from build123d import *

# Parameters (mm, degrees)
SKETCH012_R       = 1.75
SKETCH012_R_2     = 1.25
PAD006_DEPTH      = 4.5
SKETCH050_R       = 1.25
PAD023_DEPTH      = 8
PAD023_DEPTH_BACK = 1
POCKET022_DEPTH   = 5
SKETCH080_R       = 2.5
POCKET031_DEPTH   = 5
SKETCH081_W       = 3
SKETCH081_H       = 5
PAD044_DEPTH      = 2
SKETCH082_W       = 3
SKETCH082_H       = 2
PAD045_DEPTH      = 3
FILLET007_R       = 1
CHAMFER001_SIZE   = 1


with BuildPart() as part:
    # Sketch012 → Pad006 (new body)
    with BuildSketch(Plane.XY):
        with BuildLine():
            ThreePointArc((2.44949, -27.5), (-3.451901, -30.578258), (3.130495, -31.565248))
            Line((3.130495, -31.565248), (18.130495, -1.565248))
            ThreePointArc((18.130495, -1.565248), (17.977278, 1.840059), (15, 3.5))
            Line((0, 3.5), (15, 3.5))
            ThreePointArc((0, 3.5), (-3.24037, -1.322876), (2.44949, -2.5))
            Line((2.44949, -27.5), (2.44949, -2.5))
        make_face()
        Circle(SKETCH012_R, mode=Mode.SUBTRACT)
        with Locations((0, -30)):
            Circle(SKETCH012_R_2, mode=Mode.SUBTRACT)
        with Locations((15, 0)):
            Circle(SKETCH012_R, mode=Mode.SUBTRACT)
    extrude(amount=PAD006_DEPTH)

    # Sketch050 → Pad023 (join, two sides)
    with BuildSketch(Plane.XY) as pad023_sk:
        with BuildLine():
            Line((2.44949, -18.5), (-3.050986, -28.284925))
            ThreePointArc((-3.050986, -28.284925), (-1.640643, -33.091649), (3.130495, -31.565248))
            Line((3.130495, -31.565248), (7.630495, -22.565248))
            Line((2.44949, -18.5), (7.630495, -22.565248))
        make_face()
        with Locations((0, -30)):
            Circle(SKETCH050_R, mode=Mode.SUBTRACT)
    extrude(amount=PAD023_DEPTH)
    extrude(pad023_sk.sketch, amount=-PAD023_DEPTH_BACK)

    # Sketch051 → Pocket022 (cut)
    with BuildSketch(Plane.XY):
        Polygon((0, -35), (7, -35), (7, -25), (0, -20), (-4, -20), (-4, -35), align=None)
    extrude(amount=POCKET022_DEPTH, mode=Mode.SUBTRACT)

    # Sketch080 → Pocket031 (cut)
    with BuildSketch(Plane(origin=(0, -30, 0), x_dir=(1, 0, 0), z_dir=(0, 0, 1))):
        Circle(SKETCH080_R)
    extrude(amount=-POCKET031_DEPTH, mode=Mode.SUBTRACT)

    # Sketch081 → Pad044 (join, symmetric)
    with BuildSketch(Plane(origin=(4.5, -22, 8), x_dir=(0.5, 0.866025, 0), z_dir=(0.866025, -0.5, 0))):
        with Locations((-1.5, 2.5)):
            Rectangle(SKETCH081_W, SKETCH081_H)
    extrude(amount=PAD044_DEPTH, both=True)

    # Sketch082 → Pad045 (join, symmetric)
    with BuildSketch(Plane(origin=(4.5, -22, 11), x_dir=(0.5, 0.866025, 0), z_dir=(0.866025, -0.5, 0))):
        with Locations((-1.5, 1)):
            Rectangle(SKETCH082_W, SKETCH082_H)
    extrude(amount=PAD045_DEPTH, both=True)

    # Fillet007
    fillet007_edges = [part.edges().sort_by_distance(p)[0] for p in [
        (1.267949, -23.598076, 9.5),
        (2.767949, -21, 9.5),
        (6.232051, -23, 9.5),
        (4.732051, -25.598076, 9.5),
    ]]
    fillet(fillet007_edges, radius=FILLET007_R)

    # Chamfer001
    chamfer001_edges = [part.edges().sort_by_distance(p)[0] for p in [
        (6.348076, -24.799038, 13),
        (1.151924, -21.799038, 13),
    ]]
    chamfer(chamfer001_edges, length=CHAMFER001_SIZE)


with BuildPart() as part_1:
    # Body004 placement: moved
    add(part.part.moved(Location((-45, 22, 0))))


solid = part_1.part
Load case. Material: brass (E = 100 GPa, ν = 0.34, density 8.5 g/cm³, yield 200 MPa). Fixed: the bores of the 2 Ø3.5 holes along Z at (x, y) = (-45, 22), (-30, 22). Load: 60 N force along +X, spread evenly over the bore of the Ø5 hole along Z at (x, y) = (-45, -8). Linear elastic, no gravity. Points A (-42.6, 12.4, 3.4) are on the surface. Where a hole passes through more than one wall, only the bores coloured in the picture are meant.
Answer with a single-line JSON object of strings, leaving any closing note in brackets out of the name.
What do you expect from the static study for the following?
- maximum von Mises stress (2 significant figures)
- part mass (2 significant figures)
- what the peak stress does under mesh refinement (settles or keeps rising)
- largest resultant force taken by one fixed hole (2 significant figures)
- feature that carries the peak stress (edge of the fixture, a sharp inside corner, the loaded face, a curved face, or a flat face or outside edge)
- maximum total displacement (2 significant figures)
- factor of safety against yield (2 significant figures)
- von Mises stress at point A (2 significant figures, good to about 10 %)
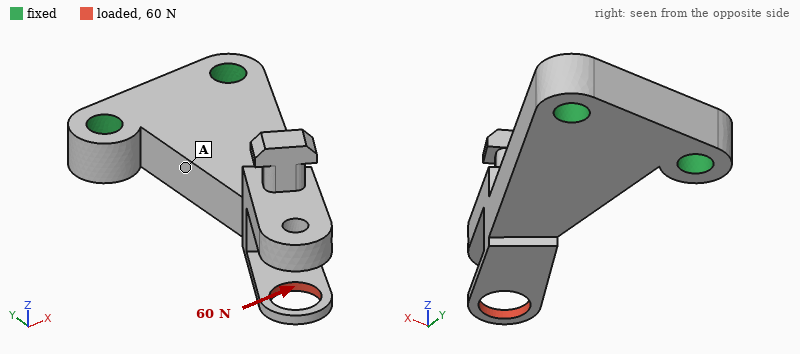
{"maximum von Mises stress": "100 MPa", "part mass": "16 g", "what the peak stress does under mesh refinement": "settles", "largest resultant force taken by one fixed hole": "130 N", "feature that carries the peak stress": "the loaded face", "maximum total displacement": "43 µm", "factor of safety against yield": "1.9", "von Mises stress at point A": "14 MPa"}
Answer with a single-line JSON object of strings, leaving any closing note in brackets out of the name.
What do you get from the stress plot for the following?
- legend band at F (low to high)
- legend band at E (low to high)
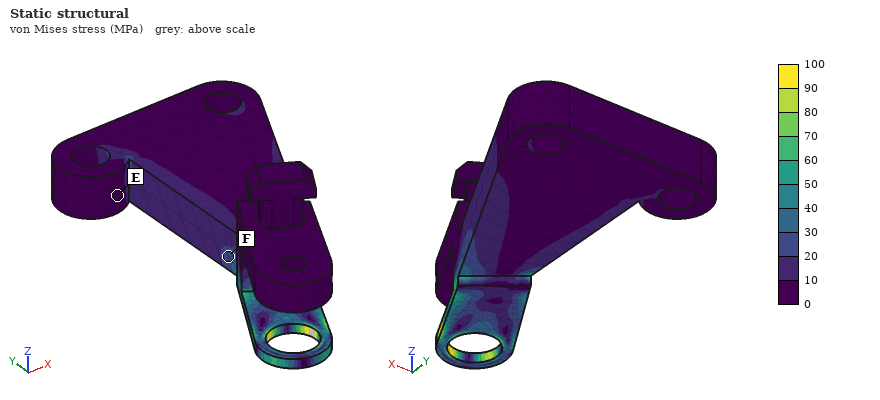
{"legend band at F": "20 to 30 MPa", "legend band at E": "0 to 10 MPa"}
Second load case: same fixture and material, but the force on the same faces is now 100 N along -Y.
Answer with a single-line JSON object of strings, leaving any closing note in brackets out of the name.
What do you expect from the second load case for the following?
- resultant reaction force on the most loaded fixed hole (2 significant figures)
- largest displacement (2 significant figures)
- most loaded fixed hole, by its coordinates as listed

{"resultant reaction force on the most loaded fixed hole": "110 N", "largest displacement": "39 µm", "most loaded fixed hole, by its coordinates as listed": "(-45, 22)"}
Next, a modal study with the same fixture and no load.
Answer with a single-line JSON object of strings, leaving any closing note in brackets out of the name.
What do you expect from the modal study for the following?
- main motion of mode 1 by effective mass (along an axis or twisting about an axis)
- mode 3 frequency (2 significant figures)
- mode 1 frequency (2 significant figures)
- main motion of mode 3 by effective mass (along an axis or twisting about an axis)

{"main motion of mode 1 by effective mass": "along Z", "mode 3 frequency": "5700 Hz", "mode 1 frequency": "2500 Hz", "main motion of mode 3 by effective mass": "along X"}
